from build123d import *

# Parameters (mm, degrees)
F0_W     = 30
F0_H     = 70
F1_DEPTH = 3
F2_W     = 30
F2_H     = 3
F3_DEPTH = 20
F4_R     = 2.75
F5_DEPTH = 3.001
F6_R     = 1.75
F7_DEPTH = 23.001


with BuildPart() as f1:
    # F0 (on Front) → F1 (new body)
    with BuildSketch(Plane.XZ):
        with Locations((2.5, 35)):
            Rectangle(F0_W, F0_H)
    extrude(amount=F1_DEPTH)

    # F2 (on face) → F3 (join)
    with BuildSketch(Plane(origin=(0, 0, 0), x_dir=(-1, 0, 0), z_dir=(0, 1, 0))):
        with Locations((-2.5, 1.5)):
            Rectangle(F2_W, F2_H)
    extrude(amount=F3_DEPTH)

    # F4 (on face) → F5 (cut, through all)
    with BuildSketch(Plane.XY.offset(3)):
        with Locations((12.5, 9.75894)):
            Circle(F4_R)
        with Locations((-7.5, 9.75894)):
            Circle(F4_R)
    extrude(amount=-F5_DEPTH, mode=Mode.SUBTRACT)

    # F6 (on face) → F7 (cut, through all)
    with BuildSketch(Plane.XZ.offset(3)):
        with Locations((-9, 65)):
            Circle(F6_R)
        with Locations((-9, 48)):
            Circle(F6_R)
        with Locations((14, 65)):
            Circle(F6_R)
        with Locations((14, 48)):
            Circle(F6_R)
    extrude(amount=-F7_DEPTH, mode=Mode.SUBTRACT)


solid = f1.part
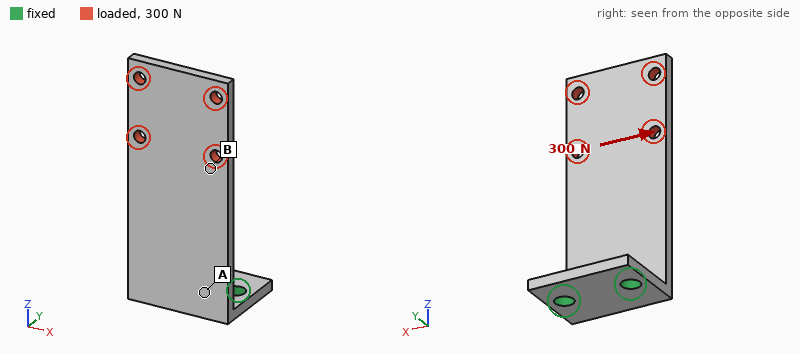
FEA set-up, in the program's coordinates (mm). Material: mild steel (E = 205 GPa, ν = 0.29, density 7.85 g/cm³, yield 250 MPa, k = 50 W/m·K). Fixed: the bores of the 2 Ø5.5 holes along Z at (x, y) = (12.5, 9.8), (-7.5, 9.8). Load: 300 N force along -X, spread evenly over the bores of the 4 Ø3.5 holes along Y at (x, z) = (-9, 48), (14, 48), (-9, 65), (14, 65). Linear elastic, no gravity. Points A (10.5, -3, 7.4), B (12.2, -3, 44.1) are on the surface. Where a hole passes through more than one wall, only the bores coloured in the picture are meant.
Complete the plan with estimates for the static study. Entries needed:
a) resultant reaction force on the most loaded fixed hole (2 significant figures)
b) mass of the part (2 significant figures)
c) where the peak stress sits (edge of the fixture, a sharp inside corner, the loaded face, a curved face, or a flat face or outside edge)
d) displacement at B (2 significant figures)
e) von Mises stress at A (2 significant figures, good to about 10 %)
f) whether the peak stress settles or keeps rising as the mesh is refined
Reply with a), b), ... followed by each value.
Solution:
a) 790 N
b) 62 g
c) edge of the fixture
d) 0.091 mm
e) 40 MPa
f) keeps rising
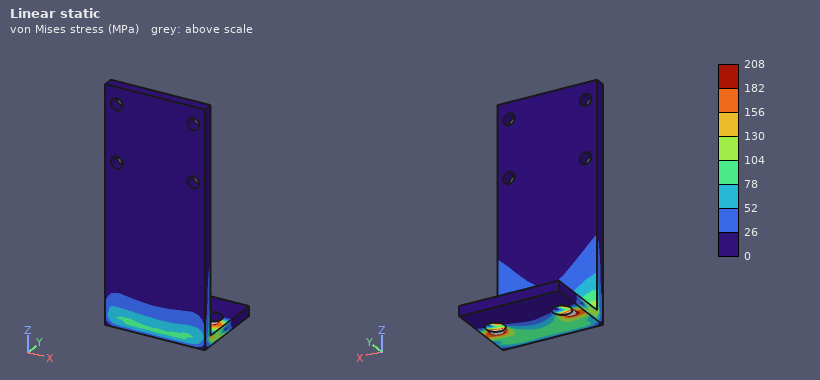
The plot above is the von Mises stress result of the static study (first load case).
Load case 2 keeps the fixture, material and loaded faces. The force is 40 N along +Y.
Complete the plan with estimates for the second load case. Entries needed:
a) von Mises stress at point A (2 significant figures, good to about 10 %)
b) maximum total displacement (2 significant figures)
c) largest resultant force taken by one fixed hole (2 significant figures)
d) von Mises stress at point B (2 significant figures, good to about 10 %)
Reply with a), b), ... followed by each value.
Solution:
a) 40 MPa
b) 0.30 mm
c) 28 N
d) 10 MPa
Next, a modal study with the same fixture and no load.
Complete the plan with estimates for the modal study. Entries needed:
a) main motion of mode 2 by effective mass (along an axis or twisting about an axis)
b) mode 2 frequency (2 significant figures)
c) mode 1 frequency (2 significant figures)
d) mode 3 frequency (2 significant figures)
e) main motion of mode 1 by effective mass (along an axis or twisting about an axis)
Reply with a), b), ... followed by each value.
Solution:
a) along X
b) 1600 Hz
c) 450 Hz
d) 2600 Hz
e) along Y
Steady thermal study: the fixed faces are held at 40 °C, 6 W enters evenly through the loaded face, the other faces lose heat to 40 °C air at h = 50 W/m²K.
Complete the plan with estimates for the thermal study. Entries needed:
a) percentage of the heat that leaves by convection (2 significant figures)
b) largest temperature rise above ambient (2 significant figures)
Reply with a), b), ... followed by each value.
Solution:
a) 74 %
b) 37 K
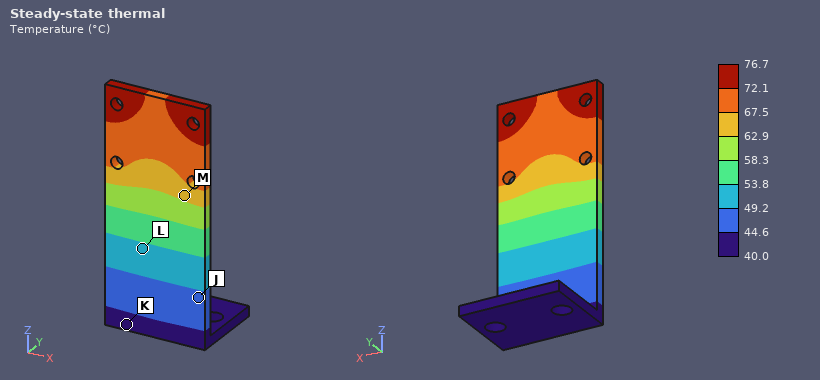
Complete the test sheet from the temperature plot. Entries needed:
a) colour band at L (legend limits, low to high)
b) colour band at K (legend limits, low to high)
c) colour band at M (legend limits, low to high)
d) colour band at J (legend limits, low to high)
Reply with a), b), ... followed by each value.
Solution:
a) 49.2 to 53.8 °C
b) 40.0 to 44.6 °C
c) 62.9 to 67.5 °C
d) 44.6 to 49.2 °C
